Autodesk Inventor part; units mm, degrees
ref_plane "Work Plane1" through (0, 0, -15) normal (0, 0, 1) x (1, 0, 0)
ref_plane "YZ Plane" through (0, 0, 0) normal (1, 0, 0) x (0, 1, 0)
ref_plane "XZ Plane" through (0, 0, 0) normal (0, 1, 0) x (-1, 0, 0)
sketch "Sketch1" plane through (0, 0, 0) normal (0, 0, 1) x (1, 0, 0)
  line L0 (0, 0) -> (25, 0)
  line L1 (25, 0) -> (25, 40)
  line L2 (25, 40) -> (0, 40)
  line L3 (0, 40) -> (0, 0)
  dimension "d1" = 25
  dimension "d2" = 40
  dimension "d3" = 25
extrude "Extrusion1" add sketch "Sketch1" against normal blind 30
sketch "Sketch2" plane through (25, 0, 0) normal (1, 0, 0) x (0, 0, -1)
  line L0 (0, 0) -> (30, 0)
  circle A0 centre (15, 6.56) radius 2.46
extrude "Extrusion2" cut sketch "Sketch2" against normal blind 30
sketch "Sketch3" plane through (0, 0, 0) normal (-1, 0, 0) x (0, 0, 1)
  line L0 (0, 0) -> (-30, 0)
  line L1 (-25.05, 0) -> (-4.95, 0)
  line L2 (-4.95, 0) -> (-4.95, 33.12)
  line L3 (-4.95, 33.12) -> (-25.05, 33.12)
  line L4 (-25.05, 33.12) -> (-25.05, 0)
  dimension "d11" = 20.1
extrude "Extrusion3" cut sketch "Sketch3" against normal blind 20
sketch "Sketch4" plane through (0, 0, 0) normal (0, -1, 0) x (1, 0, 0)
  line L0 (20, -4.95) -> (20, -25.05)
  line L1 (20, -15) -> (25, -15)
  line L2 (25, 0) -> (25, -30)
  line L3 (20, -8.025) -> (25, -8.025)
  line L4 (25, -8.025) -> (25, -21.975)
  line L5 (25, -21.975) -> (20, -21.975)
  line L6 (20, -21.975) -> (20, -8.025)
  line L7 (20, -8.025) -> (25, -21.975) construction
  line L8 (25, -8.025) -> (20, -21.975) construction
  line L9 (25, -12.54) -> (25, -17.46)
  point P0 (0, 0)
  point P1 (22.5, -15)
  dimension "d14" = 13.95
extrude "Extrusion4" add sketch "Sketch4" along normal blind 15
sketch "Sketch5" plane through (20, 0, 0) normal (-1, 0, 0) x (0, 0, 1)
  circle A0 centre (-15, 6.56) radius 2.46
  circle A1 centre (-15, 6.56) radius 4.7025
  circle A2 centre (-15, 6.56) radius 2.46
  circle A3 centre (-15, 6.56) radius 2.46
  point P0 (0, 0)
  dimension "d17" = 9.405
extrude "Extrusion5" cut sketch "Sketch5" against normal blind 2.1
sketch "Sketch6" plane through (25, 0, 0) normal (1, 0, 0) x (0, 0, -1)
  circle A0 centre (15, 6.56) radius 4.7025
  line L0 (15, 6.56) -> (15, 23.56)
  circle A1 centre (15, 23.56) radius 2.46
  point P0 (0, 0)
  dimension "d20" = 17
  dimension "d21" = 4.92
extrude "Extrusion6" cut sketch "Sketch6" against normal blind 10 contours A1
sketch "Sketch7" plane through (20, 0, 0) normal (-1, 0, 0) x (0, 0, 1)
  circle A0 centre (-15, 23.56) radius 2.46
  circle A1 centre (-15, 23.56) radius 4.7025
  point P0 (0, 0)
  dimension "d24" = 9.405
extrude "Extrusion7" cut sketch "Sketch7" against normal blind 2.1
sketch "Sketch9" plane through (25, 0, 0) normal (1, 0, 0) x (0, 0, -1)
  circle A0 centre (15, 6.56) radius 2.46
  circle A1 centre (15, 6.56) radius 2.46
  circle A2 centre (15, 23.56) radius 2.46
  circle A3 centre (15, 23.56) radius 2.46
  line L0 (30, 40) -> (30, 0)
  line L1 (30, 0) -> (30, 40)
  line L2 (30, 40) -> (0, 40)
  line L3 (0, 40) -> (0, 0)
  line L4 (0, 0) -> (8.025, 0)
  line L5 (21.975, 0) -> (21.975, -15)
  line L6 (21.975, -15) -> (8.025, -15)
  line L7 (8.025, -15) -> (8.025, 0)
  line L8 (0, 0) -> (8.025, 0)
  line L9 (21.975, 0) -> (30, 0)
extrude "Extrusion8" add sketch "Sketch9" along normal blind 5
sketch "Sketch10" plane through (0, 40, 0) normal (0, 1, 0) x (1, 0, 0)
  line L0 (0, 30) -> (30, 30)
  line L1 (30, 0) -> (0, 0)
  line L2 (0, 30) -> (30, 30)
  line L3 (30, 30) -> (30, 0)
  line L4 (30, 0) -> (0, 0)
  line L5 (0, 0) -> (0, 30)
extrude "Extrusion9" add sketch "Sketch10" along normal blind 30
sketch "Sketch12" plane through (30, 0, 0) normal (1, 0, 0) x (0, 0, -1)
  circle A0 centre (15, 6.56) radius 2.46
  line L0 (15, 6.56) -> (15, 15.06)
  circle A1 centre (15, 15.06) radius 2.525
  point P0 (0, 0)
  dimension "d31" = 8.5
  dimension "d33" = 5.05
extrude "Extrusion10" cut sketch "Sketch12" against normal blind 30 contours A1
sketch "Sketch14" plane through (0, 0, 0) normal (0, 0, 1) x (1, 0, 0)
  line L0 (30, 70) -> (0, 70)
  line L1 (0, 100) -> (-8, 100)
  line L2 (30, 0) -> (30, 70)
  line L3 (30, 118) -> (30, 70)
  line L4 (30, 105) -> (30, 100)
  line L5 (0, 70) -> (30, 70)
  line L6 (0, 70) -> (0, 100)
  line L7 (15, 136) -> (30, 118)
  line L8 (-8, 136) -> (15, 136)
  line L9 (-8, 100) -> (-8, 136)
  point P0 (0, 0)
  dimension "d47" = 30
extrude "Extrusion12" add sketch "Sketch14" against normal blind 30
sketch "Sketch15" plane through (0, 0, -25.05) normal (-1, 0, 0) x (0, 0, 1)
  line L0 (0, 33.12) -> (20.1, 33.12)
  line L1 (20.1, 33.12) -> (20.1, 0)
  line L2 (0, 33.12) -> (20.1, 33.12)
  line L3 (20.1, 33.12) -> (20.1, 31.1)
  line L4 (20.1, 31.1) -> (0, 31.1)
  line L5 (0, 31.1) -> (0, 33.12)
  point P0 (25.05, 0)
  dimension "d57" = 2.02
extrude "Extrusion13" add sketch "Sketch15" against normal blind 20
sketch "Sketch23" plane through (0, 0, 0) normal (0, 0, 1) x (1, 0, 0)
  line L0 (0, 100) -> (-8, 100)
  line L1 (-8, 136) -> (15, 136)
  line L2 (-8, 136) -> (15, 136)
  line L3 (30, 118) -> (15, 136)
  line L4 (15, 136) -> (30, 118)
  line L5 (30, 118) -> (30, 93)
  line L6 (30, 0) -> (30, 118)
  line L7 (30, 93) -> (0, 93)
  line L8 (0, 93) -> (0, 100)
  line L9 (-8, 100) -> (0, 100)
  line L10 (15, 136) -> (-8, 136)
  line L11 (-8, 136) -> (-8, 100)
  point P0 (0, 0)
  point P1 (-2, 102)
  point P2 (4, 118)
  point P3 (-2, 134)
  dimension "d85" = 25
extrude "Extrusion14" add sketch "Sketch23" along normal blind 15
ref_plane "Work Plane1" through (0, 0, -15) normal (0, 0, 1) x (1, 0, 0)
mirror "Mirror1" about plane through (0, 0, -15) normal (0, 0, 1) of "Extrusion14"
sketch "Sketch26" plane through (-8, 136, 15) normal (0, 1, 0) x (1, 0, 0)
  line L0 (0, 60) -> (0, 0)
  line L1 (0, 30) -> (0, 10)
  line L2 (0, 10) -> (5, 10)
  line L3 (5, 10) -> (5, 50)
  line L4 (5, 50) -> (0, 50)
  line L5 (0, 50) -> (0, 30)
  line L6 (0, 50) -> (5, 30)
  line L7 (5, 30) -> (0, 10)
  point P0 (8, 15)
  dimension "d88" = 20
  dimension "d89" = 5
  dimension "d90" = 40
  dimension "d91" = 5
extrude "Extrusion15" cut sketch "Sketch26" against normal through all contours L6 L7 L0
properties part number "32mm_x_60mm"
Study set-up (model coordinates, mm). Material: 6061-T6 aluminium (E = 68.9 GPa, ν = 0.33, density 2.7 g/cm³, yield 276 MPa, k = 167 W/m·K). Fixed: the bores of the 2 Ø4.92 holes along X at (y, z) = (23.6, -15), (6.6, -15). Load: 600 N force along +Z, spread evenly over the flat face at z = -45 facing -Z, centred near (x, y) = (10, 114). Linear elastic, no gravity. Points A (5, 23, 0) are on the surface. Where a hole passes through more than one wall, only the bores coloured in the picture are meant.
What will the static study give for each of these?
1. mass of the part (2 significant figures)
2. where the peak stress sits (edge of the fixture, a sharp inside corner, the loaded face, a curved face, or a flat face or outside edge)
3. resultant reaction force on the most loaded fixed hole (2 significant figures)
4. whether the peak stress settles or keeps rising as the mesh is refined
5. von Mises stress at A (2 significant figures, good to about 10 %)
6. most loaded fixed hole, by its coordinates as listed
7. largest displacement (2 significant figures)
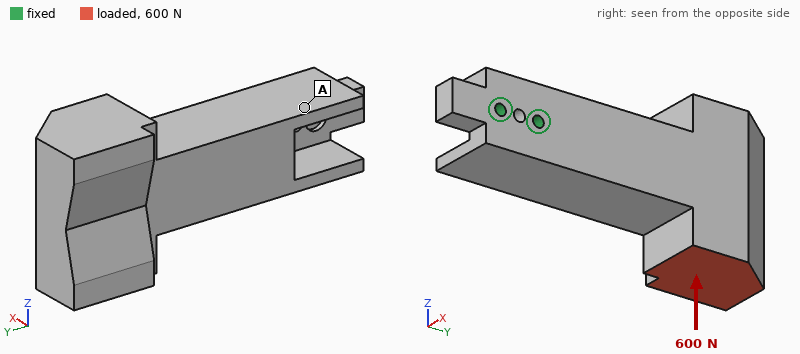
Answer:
420 g
edge of the fixture
2.9 kN
keeps rising
8.9 MPa
(23.6, -15)
0.14 mm
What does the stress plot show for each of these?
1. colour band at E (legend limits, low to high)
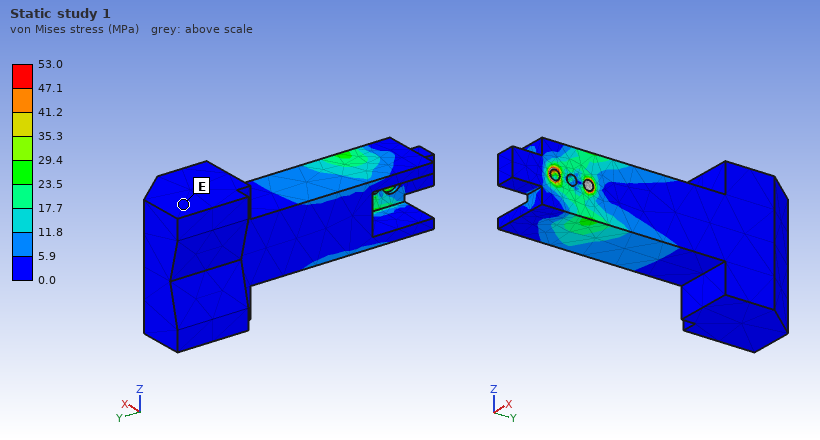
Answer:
0.0 to 5.9 MPa
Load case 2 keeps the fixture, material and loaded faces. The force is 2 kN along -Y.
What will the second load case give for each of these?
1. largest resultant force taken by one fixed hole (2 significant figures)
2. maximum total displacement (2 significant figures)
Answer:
3.1 kN
0.21 mm
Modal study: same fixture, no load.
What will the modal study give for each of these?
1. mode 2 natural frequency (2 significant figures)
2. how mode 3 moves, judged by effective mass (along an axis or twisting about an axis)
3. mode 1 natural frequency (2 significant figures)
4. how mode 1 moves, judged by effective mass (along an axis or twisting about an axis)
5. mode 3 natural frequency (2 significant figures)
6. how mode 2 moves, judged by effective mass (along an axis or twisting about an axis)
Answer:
750 Hz
twisting about Y
650 Hz
along X
1800 Hz
along Z
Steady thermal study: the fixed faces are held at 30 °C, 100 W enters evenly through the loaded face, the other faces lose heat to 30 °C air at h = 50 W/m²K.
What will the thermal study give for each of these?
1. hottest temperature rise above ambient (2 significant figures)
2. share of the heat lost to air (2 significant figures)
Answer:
60 K
37 %
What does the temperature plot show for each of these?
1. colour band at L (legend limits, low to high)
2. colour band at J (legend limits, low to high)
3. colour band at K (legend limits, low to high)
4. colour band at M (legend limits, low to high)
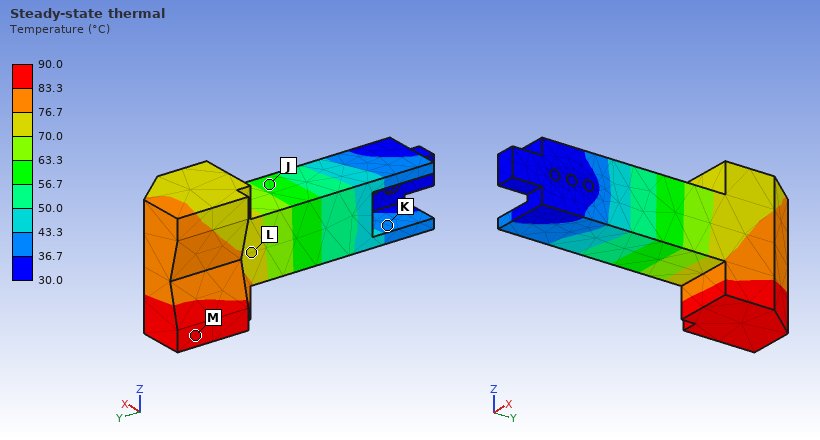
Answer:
70.0 to 76.7 °C
56.7 to 63.3 °C
36.7 to 43.3 °C
83.3 to 90.0 °C
